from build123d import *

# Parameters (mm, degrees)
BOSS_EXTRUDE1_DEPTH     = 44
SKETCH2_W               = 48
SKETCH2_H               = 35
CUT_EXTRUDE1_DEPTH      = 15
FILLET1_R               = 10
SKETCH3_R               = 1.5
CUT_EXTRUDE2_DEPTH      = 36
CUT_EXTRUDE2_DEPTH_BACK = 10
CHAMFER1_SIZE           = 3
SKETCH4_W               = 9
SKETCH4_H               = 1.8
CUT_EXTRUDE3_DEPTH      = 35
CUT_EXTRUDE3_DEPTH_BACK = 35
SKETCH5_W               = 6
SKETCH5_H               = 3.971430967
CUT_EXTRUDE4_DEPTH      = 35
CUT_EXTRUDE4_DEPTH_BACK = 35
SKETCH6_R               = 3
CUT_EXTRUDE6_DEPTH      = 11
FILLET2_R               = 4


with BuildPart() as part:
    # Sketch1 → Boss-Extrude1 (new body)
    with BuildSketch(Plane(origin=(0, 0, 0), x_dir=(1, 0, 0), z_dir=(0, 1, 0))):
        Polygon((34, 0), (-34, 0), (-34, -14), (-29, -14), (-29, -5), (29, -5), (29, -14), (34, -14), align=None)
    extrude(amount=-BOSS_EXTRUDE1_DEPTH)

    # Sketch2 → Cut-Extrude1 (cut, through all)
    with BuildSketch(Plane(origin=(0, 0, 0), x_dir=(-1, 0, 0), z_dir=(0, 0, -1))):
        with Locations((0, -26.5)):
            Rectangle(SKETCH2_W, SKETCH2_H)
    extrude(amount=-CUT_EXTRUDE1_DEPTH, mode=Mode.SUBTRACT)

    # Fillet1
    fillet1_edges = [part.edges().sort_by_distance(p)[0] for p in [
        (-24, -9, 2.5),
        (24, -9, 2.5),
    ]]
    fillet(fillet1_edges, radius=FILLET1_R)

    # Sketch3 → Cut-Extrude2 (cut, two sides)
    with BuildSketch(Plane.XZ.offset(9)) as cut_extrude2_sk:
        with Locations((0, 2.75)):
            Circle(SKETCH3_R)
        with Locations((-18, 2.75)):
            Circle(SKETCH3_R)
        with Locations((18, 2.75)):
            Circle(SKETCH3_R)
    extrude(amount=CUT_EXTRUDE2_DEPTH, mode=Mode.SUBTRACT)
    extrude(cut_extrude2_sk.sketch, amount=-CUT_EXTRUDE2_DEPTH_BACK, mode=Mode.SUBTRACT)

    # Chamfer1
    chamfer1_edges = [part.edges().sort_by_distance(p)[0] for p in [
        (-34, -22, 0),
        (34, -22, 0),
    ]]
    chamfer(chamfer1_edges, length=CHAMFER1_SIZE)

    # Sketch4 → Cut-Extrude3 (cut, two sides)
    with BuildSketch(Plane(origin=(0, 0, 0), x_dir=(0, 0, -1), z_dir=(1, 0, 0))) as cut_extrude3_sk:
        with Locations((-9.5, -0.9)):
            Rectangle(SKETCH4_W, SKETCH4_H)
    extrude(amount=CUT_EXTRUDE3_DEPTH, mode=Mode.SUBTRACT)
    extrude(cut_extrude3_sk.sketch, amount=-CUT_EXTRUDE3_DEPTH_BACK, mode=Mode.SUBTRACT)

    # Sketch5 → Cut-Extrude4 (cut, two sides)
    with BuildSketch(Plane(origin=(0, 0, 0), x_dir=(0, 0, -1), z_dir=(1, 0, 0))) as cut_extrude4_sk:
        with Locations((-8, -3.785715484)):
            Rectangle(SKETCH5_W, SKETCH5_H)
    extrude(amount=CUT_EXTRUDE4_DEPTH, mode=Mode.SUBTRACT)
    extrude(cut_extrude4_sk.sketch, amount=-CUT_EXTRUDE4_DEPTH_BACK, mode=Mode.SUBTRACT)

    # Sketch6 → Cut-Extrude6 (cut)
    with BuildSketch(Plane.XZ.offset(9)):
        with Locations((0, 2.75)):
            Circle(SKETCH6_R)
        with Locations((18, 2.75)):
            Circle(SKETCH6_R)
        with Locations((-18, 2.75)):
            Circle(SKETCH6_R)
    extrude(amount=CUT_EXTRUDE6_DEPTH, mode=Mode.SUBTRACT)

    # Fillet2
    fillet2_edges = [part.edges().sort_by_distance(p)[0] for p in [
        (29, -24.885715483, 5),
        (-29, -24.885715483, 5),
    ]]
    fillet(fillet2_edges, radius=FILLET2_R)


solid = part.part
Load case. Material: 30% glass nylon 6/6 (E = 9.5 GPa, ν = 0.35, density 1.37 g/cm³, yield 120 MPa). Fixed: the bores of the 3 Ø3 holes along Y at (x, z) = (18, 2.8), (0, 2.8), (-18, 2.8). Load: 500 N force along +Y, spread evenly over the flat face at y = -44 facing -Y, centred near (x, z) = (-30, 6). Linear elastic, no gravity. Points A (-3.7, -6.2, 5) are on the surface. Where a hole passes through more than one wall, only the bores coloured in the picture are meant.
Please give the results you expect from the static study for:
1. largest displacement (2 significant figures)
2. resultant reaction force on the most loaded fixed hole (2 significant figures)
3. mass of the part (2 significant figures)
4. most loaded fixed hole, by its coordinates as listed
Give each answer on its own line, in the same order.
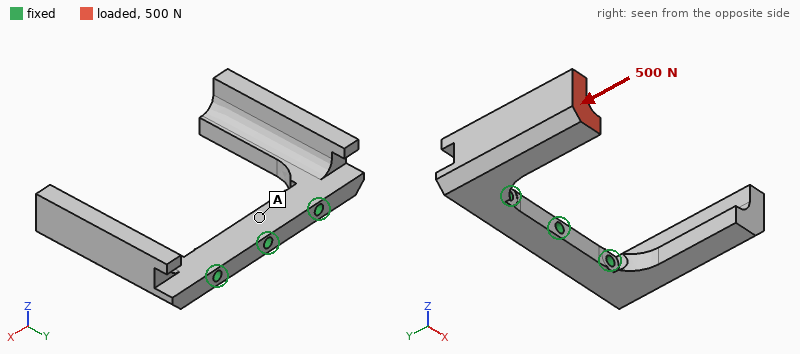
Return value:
0.75 mm
510 N
14 g
(-18, 2.8)
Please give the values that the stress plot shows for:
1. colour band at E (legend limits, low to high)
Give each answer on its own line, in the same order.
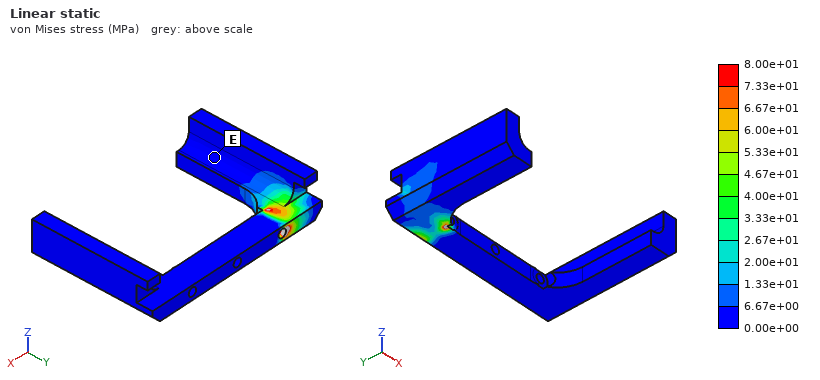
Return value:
0.00e+00 to 6.67e+00 MPa
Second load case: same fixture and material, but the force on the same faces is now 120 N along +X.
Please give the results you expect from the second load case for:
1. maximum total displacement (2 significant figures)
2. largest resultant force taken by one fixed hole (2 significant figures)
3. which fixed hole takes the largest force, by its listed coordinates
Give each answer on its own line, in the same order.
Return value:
0.87 mm
120 N
(-18, 2.8)
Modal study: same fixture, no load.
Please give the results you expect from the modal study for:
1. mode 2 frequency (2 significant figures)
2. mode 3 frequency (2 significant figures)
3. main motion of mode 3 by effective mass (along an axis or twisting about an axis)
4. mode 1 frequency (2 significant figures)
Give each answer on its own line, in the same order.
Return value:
1000 Hz
1600 Hz
along X
1000 Hz
